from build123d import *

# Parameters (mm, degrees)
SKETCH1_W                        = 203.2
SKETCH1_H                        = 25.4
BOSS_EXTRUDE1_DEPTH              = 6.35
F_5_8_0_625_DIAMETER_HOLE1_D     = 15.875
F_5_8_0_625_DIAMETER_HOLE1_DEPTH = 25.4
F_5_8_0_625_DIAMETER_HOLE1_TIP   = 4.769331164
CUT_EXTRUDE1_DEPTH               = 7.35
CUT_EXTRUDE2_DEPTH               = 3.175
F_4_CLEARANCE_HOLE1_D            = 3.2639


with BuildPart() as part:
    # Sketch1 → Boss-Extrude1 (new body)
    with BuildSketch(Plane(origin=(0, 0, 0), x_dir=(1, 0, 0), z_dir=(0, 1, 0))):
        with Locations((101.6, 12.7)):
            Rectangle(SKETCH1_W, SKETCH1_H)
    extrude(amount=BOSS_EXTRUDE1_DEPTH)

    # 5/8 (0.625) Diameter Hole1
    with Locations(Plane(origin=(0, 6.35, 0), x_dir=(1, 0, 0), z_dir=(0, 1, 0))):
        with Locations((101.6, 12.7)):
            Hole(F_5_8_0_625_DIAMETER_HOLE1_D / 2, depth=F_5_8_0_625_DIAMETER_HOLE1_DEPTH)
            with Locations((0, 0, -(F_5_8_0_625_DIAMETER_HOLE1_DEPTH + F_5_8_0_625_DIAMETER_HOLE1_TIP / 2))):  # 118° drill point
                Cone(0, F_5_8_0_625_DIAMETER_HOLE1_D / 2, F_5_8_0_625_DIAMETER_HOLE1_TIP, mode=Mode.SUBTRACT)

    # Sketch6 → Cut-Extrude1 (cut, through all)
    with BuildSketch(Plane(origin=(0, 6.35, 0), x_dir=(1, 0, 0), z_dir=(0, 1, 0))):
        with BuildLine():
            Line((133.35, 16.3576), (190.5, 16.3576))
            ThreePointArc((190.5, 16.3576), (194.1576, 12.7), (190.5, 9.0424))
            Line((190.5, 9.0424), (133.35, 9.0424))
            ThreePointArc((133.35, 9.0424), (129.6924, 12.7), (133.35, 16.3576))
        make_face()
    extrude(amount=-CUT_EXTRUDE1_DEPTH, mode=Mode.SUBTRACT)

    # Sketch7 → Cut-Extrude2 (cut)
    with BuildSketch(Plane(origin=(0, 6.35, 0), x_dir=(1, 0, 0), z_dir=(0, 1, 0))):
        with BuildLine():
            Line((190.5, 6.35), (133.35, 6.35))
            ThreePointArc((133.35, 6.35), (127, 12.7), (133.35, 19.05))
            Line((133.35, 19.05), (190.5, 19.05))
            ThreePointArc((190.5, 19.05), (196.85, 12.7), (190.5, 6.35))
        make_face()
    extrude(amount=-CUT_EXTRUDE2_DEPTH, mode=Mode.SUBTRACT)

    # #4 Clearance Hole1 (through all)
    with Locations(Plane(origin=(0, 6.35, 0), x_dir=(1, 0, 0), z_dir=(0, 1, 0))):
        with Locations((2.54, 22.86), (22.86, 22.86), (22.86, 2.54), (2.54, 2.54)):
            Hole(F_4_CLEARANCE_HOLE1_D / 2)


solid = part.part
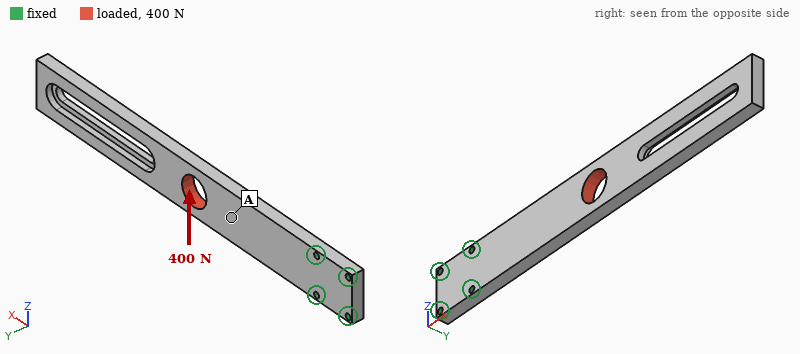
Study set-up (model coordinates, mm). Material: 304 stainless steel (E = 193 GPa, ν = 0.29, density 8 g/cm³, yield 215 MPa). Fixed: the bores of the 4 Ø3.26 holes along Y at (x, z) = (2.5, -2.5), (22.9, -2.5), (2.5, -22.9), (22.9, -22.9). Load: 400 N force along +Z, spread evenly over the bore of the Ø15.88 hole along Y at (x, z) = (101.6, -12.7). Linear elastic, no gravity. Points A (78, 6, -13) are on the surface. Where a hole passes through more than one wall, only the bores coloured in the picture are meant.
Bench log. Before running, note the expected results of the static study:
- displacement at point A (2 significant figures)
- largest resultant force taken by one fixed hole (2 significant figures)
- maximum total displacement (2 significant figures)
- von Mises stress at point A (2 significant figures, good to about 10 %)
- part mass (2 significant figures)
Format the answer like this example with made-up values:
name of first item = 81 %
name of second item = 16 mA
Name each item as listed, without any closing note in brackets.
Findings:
displacement at point A = 0.023 mm
largest resultant force taken by one fixed hole = 1.5 kN
maximum total displacement = 0.12 mm
von Mises stress at point A = 6.8 MPa
part mass = 220 g
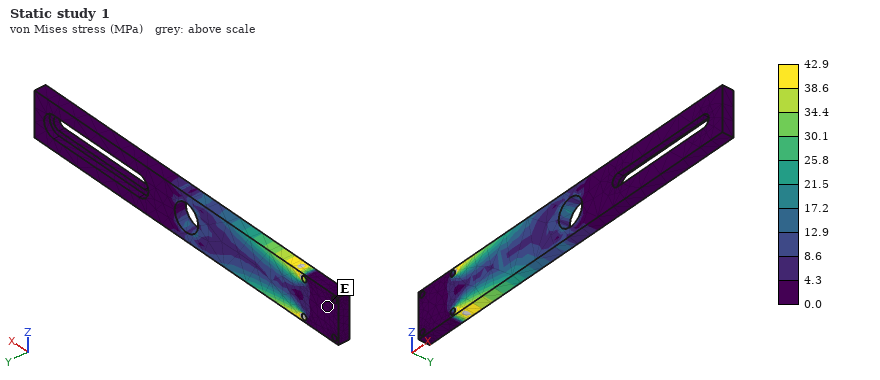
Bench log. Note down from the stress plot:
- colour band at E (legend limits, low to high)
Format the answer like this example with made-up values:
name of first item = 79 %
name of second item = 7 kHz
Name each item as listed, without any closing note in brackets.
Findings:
colour band at E = 0.0 to 4.3 MPa
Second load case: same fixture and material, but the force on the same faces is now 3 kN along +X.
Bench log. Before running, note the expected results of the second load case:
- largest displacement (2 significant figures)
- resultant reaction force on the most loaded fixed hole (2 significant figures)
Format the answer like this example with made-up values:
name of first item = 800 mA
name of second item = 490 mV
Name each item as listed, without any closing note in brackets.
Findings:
largest displacement = 10 µm
resultant reaction force on the most loaded fixed hole = 1.3 kN
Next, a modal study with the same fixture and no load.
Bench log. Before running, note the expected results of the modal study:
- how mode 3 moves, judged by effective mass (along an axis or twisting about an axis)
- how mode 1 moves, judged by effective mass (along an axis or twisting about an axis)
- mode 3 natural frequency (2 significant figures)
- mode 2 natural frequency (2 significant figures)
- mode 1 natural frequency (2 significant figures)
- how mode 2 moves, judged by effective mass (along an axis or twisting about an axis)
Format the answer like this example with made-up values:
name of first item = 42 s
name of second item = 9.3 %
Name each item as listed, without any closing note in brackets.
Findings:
how mode 3 moves, judged by effective mass = along Y
how mode 1 moves, judged by effective mass = along Y
mode 3 natural frequency = 910 Hz
mode 2 natural frequency = 680 Hz
mode 1 natural frequency = 170 Hz
how mode 2 moves, judged by effective mass = along Z
